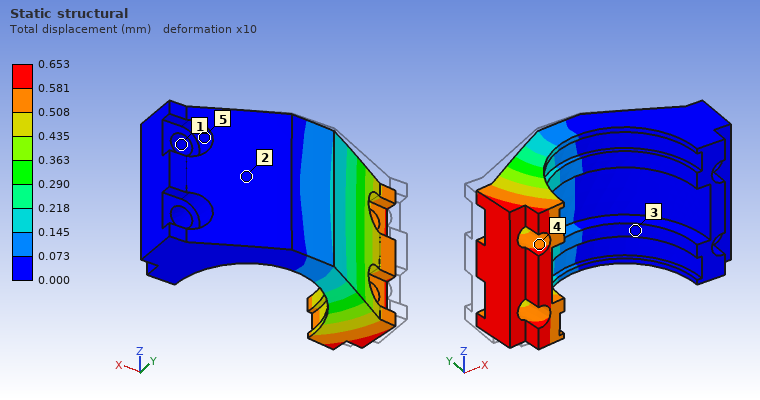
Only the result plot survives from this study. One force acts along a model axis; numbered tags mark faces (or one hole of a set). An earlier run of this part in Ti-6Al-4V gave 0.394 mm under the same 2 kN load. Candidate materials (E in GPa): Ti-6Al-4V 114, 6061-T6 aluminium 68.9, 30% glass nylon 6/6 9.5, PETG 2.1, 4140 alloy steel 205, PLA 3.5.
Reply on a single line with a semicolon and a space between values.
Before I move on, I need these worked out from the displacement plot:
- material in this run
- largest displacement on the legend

6061-T6 aluminium; 0.653 mm
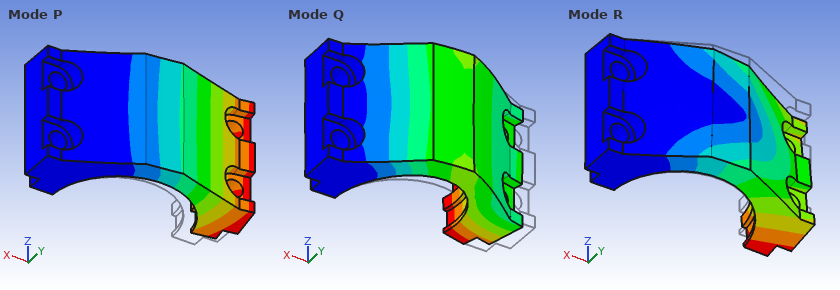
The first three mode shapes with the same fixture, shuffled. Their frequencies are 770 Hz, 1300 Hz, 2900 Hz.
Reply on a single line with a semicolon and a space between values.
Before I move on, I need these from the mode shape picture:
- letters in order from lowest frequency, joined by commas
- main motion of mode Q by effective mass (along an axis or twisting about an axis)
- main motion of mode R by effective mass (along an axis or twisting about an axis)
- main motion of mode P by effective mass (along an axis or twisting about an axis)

P, R, Q; along X; along Z; along Y
